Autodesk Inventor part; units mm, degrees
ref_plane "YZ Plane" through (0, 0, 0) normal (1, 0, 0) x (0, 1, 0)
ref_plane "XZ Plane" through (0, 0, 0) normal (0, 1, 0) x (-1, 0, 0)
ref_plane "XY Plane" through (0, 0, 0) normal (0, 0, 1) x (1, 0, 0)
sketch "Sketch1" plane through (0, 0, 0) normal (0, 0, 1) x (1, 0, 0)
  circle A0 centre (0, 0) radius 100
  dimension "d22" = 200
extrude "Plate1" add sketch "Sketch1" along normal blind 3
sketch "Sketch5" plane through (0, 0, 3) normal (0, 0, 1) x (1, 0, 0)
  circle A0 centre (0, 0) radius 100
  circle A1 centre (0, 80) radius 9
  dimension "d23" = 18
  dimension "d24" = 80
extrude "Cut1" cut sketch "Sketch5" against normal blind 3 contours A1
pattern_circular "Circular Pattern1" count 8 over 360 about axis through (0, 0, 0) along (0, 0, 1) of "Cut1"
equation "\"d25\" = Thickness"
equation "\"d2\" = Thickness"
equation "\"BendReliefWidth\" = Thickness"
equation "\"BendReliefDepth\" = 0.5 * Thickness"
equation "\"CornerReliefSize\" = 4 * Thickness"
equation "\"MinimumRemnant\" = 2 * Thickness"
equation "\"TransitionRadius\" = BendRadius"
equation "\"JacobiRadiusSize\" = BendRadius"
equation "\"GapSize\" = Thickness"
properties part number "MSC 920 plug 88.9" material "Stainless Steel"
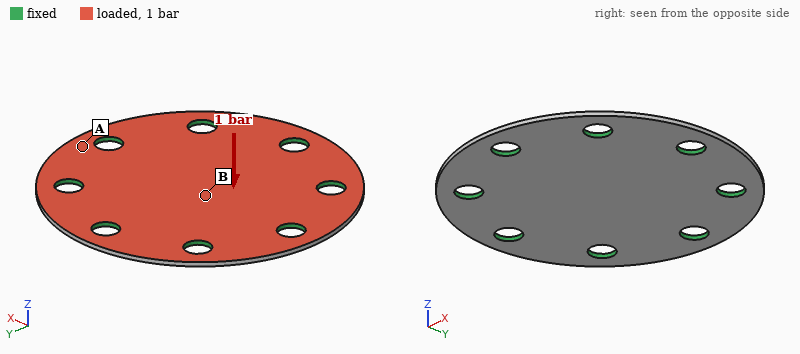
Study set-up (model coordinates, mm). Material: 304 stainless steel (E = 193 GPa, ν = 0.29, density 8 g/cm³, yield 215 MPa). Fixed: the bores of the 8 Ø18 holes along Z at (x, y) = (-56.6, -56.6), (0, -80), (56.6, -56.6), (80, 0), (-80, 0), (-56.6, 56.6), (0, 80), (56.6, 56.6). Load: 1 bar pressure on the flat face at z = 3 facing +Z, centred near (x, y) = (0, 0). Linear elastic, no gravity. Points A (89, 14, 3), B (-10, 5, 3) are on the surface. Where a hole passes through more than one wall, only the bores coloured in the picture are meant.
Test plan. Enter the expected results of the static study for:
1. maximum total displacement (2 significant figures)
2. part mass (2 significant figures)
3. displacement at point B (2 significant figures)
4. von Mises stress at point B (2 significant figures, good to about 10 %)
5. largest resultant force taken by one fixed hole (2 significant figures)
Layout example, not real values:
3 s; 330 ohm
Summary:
0.10 mm; 710 g; 0.099 mm; 28 MPa; 370 N
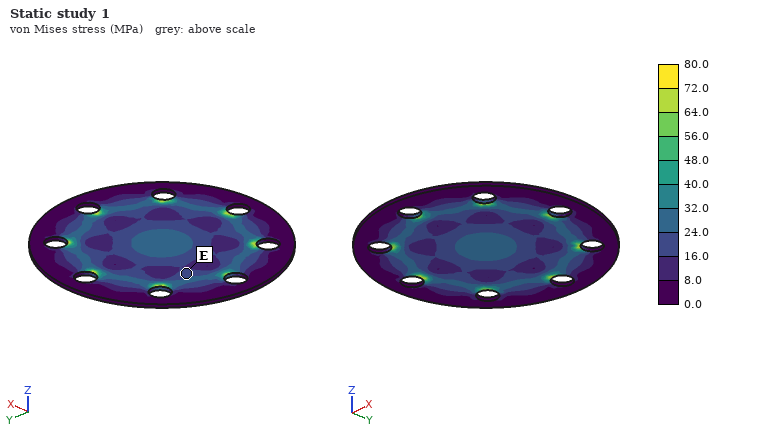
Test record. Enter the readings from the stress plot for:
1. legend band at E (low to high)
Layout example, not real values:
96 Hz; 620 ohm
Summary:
16.0 to 24.0 MPa
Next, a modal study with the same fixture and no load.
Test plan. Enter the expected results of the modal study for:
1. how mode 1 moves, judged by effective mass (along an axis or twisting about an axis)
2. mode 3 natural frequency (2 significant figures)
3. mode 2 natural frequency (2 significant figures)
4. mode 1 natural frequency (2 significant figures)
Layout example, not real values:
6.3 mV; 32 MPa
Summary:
along Z; 2600 Hz; 2600 Hz; 1300 Hz
